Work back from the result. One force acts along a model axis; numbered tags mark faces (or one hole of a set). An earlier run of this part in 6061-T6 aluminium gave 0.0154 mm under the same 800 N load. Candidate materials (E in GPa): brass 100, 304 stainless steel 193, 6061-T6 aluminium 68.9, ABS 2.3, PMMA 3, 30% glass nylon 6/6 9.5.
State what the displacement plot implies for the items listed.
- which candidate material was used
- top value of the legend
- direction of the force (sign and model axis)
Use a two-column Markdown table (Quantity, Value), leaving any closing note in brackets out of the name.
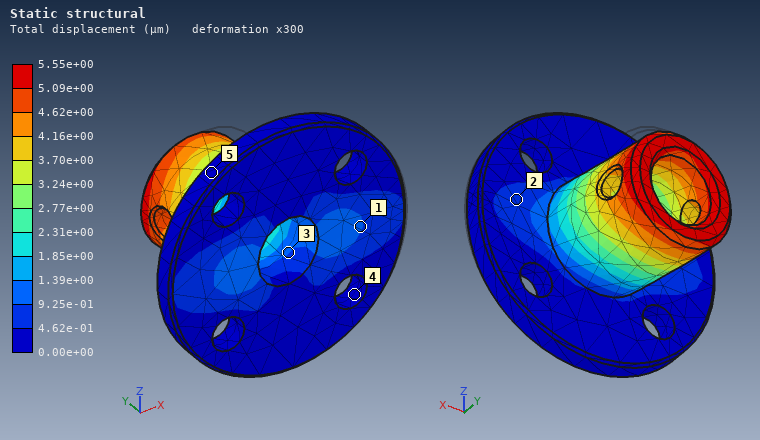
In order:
| Quantity | Value |
|---|---|
| which candidate material was used | 304 stainless steel |
| top value of the legend | 5.55e+00 µm |
| direction of the force | -X |
